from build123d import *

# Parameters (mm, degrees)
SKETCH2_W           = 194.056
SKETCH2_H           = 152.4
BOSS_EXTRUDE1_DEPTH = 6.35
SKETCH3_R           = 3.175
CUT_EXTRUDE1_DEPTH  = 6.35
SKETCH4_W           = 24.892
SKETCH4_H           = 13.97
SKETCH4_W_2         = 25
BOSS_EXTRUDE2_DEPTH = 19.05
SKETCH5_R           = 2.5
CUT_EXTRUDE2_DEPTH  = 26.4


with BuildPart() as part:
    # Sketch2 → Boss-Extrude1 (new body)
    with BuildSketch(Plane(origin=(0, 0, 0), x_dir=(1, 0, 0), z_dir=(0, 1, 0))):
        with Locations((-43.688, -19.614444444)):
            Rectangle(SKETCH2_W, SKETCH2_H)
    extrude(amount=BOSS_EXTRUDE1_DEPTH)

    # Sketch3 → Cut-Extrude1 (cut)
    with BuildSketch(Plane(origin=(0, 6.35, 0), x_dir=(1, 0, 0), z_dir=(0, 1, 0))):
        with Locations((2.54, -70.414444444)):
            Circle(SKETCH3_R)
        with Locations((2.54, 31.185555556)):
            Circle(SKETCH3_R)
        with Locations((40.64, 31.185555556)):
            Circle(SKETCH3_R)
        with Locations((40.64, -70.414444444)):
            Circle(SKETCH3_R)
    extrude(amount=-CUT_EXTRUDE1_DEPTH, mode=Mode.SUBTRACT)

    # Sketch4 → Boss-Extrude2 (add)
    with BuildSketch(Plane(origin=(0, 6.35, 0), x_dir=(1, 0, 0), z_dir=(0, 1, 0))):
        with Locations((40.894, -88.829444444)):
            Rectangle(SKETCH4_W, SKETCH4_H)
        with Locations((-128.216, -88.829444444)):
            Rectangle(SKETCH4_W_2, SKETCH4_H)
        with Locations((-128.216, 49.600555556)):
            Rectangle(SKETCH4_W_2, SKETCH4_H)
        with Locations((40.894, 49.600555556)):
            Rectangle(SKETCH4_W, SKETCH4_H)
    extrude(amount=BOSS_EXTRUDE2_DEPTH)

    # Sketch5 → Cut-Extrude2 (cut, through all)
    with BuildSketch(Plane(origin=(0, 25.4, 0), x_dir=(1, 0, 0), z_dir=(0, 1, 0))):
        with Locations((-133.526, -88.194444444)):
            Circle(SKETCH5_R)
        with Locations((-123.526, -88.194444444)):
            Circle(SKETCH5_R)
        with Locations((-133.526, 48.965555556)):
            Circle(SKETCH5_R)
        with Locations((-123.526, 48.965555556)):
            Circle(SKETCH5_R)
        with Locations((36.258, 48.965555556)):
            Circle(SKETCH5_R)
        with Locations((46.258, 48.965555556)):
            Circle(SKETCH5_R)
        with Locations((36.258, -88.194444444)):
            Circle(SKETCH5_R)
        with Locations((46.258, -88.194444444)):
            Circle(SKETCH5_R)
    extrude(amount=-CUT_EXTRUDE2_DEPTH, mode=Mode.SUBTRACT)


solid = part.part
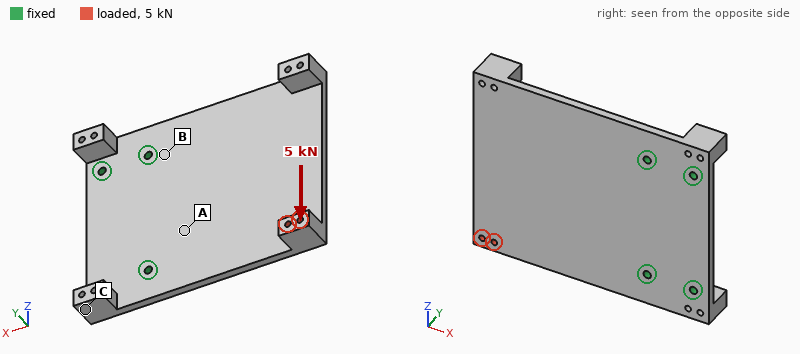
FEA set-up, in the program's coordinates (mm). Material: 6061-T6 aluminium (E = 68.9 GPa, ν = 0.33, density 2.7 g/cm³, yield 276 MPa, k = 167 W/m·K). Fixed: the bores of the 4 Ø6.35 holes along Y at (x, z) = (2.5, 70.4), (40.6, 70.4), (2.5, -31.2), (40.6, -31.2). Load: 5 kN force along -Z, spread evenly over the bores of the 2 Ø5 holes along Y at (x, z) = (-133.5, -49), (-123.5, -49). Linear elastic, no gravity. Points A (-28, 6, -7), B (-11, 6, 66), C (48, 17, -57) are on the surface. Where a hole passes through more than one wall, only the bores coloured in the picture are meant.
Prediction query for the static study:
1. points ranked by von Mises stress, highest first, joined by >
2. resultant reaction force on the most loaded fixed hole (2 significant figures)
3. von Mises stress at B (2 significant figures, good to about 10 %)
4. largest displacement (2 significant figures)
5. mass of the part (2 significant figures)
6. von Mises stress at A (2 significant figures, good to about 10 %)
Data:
A > B > C
5.4 kN
29 MPa
1.5 mm
570 g
44 MPa
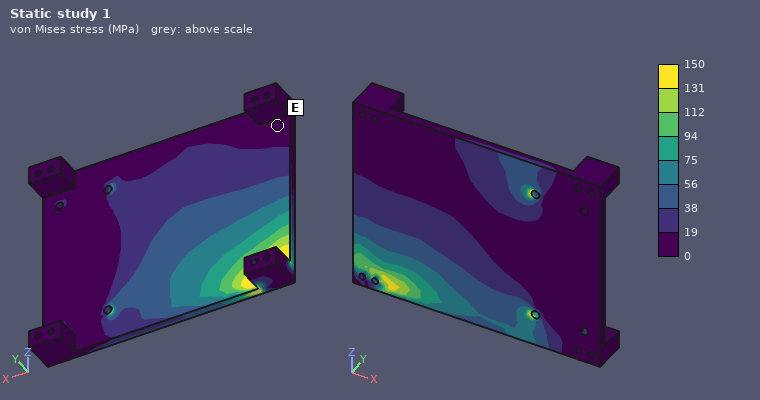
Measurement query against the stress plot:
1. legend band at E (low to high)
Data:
0 to 19 MPa
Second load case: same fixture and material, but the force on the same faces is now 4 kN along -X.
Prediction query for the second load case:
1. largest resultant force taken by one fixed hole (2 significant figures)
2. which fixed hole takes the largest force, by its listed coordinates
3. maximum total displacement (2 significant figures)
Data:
3.4 kN
(2.5, -31.2)
2.5 mm
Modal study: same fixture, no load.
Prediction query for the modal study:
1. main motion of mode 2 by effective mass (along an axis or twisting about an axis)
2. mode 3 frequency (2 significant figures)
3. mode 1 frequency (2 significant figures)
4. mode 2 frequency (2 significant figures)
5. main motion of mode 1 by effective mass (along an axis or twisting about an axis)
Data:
twisting about X
1400 Hz
220 Hz
470 Hz
along Y
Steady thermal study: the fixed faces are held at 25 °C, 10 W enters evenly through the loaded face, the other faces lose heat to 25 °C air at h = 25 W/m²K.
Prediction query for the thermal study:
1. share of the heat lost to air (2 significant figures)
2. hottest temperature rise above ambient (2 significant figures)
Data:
45 %
14 K
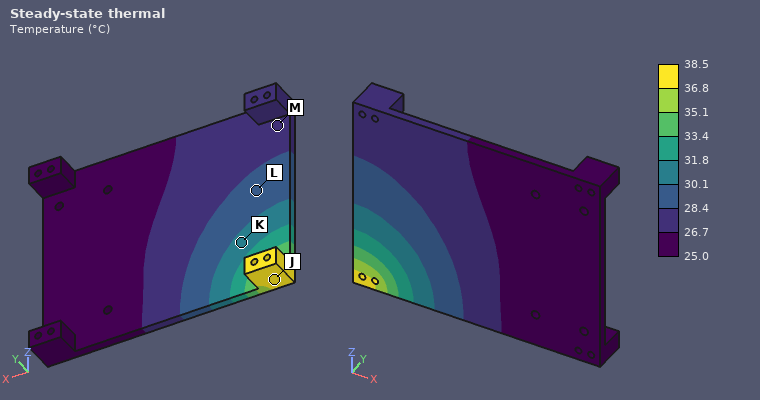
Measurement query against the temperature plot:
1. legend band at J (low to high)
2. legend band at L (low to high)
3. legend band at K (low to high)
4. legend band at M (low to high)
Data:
36.8 to 38.5 °C
28.4 to 30.1 °C
30.1 to 31.8 °C
26.7 to 28.4 °C
